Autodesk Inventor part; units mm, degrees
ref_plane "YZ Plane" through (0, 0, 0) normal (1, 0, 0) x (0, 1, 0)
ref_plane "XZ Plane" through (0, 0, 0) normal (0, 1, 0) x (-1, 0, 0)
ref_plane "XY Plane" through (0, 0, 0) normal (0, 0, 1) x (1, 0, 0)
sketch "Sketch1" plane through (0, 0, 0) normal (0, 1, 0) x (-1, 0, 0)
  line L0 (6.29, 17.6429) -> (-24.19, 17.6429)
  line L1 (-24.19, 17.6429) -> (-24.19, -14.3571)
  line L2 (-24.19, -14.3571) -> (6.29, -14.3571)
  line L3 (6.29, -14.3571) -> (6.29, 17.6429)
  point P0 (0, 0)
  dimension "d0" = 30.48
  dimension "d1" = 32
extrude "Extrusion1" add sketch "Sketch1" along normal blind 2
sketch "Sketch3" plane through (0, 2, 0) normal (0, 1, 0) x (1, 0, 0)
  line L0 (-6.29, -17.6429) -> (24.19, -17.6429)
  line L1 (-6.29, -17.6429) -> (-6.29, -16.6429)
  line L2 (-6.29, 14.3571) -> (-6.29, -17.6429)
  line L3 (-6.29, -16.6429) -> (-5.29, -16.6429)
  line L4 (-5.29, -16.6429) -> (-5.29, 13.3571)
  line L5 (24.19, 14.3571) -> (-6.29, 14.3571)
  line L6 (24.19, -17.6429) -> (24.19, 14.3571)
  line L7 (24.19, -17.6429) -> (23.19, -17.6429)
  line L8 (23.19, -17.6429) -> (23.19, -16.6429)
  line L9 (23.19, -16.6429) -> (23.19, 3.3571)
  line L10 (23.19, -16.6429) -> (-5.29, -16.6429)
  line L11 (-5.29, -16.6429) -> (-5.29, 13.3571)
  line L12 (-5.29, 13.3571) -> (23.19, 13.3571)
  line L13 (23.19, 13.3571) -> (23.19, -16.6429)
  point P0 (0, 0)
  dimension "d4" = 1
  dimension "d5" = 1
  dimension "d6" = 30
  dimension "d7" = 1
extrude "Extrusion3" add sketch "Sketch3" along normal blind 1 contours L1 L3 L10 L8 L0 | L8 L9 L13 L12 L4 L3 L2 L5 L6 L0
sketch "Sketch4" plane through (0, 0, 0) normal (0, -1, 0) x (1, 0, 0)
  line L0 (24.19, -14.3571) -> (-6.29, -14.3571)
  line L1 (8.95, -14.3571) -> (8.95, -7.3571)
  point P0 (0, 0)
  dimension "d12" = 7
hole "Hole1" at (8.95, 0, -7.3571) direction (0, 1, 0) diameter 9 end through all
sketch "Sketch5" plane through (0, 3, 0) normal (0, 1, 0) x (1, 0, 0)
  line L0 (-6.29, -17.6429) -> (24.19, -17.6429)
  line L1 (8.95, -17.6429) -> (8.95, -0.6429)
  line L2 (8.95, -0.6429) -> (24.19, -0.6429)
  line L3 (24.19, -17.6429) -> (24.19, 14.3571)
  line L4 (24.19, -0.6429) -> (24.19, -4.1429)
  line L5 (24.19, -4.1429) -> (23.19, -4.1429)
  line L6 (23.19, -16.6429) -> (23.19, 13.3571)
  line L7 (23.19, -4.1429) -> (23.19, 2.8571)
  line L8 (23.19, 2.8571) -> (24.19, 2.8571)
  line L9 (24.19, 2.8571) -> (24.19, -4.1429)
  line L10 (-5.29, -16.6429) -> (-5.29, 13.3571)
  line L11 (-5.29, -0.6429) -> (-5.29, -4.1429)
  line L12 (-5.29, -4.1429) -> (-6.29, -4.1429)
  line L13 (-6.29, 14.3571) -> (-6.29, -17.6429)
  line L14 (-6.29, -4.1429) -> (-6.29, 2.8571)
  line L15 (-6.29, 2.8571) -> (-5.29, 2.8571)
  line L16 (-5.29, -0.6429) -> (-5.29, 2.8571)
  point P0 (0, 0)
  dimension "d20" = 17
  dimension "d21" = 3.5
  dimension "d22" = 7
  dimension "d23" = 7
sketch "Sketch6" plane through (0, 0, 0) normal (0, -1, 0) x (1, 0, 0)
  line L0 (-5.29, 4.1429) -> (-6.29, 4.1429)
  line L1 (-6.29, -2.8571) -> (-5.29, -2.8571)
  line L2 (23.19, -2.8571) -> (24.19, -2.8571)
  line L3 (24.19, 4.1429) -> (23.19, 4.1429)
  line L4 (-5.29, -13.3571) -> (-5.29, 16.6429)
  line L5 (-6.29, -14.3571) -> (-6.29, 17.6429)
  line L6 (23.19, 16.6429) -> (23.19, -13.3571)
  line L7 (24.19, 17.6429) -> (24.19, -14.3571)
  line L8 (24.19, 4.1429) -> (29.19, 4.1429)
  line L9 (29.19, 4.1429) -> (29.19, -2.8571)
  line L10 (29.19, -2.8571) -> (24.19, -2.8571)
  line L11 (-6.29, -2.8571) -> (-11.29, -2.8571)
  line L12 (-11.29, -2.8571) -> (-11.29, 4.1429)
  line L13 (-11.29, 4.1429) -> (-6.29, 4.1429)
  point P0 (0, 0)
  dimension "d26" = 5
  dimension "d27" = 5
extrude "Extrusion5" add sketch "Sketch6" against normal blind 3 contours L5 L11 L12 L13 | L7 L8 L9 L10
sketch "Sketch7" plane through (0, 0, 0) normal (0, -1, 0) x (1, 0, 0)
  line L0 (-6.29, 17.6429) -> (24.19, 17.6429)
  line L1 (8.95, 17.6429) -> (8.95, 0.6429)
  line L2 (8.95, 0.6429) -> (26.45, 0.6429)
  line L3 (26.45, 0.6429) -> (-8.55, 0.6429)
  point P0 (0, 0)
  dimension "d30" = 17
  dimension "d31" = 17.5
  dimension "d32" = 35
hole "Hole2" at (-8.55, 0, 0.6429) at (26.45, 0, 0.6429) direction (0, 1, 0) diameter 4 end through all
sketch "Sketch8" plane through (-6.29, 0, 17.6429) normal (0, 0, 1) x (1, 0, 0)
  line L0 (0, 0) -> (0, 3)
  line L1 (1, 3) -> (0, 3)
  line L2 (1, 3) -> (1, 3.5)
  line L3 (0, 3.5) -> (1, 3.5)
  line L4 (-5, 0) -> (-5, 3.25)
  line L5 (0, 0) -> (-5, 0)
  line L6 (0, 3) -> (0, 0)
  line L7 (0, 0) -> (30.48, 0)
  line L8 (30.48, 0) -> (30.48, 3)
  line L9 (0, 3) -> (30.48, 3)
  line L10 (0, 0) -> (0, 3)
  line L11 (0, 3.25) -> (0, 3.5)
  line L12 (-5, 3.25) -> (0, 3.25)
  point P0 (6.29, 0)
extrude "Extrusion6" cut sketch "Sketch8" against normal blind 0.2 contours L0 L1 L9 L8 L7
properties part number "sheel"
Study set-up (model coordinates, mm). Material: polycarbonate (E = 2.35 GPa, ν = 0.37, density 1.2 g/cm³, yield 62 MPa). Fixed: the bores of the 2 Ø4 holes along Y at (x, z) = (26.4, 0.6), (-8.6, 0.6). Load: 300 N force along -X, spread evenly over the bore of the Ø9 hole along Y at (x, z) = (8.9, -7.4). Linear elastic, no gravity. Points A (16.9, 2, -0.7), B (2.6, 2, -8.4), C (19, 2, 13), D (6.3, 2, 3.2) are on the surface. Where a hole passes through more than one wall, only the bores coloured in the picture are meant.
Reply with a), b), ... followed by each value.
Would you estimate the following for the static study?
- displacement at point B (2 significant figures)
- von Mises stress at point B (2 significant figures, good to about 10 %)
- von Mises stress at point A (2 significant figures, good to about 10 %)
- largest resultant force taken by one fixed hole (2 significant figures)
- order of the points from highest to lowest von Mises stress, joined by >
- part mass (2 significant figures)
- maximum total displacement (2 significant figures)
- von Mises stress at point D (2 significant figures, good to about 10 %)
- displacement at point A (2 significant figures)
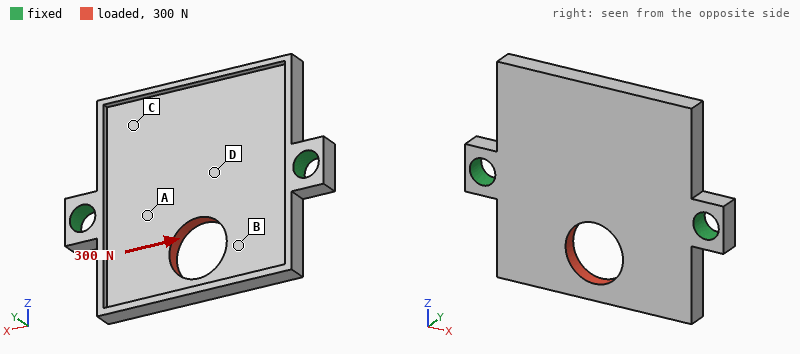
a) 0.089 mm
b) 11 MPa
c) 7.1 MPa
d) 170 N
e) B > A > D > C
f) 2.5 g
g) 0.14 mm
h) 4.2 MPa
i) 0.027 mm
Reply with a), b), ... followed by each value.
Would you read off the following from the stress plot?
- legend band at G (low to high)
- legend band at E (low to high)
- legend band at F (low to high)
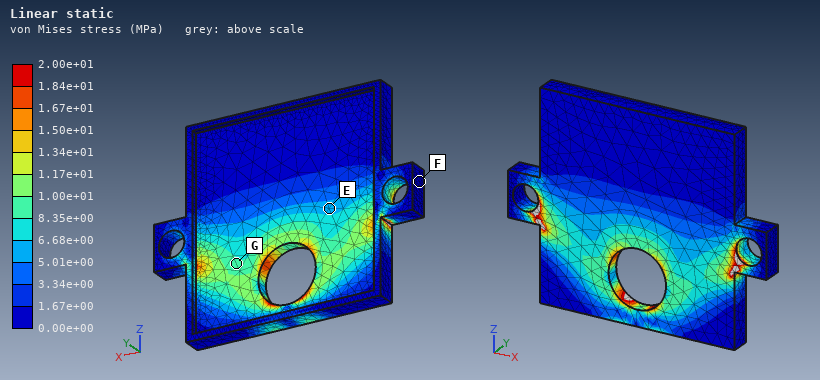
a) 8.35e+00 to 1.00e+01 MPa
b) 5.01e+00 to 6.68e+00 MPa
c) 0.00e+00 to 1.67e+00 MPa
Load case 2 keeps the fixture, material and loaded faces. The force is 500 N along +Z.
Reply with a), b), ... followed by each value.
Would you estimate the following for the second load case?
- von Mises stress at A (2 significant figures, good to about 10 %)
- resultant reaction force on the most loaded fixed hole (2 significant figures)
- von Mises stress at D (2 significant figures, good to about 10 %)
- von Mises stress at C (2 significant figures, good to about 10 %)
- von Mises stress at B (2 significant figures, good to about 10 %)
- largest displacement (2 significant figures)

a) 7.7 MPa
b) 250 N
c) 8.0 MPa
d) 5.7 MPa
e) 18 MPa
f) 0.23 mm
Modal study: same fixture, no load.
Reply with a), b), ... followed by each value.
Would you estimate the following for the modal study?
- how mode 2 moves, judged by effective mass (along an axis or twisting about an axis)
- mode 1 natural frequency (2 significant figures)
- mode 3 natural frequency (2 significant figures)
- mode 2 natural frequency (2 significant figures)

a) along Y
b) 1300 Hz
c) 2700 Hz
d) 1700 Hz
